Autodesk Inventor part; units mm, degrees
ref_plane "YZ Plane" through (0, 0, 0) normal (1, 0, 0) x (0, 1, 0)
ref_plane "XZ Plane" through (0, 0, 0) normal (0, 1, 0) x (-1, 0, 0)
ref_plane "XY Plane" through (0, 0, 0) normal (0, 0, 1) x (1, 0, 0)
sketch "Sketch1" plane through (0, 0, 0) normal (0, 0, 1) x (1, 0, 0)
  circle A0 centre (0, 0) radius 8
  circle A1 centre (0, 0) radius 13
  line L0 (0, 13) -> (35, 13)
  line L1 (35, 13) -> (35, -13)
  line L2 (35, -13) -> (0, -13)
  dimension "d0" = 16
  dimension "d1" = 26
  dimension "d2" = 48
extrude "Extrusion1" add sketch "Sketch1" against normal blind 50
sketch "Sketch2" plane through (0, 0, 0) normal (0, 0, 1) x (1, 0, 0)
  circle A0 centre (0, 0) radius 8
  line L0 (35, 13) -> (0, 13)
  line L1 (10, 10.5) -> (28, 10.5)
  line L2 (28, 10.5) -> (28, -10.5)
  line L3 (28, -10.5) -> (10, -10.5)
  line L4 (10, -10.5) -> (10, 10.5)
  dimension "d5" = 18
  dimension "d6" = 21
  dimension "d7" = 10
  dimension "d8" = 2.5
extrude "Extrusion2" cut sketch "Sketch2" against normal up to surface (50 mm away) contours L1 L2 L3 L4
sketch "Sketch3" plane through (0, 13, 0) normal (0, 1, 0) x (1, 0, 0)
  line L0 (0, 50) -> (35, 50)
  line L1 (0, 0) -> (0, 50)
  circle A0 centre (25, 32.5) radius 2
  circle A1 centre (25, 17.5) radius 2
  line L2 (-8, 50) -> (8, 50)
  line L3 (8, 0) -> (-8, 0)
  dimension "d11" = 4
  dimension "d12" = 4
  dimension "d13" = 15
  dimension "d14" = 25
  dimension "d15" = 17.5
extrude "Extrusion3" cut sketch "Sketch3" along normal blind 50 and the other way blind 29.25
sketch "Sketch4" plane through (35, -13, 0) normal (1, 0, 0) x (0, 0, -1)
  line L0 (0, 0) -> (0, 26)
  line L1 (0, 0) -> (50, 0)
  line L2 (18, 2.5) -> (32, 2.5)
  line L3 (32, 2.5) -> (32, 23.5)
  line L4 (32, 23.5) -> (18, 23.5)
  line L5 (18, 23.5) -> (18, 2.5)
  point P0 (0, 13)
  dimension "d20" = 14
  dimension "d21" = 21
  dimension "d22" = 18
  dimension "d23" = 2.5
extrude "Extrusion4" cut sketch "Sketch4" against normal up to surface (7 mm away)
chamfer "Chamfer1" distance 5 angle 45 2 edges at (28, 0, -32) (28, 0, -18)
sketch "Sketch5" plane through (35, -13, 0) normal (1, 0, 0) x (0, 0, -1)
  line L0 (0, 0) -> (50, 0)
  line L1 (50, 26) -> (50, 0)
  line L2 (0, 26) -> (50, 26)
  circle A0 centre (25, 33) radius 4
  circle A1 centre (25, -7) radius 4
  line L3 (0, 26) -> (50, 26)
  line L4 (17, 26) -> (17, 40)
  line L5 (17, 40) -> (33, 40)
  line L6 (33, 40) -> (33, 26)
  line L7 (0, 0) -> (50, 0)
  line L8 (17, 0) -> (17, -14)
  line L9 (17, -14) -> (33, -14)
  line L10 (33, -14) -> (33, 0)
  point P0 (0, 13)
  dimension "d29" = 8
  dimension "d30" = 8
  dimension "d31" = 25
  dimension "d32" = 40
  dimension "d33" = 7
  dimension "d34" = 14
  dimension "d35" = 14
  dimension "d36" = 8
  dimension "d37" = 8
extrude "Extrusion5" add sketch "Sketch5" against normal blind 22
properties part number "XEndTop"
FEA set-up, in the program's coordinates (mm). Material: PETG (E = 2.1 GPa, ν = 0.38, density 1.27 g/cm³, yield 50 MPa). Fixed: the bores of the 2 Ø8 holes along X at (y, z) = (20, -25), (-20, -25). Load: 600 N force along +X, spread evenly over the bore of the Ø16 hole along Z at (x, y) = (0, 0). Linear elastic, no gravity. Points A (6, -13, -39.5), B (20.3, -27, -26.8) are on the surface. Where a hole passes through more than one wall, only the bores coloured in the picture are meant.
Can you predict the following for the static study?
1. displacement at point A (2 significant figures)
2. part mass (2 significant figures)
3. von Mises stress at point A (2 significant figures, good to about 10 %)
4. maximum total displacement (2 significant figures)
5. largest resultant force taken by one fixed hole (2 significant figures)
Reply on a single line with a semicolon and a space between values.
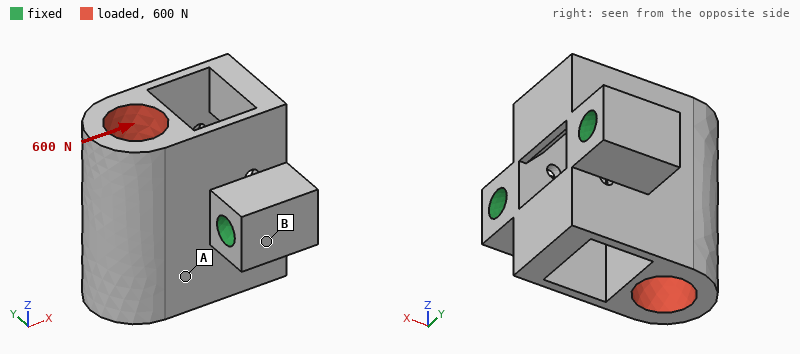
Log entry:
30 µm; 44 g; 1.7 MPa; 54 µm; 310 N
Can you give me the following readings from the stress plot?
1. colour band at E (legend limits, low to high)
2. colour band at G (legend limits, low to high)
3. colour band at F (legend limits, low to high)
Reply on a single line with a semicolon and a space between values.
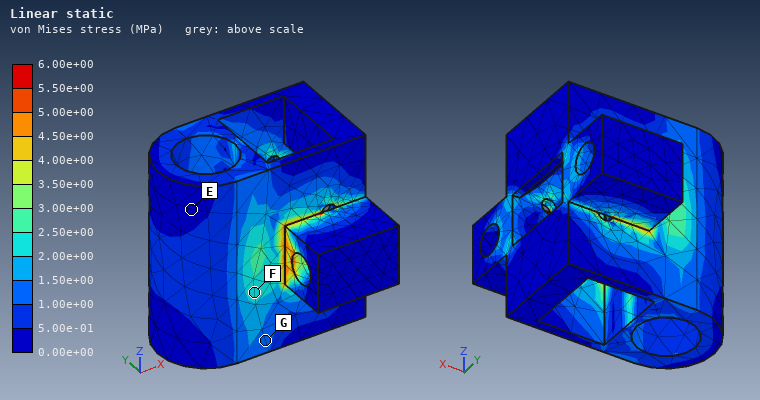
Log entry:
0.00e+00 to 5.00e-01 MPa; 1.00e+00 to 1.50e+00 MPa; 2.00e+00 to 2.50e+00 MPa
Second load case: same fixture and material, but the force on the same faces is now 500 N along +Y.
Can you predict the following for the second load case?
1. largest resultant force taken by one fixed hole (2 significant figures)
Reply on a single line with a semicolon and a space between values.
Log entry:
350 N
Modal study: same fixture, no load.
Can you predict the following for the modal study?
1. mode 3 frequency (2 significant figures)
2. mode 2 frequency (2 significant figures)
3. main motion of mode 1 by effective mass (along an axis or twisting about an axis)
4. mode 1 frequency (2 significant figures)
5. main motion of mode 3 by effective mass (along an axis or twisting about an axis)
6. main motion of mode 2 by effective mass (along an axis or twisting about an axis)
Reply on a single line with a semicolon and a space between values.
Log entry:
2400 Hz; 1900 Hz; along Z; 1600 Hz; twisting about X; along Y
